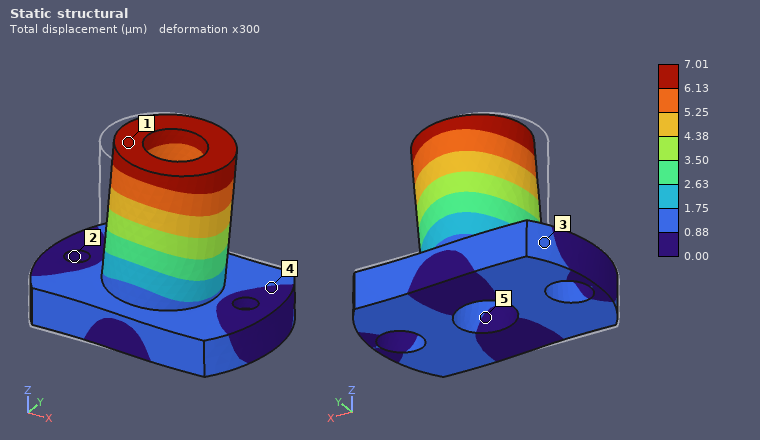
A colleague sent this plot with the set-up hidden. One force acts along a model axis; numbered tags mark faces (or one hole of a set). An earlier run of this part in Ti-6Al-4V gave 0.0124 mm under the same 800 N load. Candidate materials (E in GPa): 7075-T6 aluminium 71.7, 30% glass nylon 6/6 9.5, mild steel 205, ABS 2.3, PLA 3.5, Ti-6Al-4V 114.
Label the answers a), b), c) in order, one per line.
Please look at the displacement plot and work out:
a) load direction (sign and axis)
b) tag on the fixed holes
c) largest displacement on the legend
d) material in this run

a) +X
b) 2
c) 7.01 µm
d) mild steel
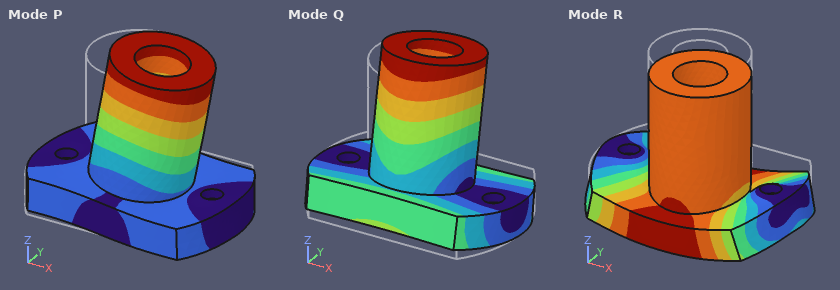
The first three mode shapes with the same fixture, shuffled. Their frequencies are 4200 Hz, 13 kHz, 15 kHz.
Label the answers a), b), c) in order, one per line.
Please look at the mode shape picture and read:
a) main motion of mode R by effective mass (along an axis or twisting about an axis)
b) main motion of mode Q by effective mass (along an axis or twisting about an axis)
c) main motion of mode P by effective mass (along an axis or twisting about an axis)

a) along Z
b) along Y
c) along X
